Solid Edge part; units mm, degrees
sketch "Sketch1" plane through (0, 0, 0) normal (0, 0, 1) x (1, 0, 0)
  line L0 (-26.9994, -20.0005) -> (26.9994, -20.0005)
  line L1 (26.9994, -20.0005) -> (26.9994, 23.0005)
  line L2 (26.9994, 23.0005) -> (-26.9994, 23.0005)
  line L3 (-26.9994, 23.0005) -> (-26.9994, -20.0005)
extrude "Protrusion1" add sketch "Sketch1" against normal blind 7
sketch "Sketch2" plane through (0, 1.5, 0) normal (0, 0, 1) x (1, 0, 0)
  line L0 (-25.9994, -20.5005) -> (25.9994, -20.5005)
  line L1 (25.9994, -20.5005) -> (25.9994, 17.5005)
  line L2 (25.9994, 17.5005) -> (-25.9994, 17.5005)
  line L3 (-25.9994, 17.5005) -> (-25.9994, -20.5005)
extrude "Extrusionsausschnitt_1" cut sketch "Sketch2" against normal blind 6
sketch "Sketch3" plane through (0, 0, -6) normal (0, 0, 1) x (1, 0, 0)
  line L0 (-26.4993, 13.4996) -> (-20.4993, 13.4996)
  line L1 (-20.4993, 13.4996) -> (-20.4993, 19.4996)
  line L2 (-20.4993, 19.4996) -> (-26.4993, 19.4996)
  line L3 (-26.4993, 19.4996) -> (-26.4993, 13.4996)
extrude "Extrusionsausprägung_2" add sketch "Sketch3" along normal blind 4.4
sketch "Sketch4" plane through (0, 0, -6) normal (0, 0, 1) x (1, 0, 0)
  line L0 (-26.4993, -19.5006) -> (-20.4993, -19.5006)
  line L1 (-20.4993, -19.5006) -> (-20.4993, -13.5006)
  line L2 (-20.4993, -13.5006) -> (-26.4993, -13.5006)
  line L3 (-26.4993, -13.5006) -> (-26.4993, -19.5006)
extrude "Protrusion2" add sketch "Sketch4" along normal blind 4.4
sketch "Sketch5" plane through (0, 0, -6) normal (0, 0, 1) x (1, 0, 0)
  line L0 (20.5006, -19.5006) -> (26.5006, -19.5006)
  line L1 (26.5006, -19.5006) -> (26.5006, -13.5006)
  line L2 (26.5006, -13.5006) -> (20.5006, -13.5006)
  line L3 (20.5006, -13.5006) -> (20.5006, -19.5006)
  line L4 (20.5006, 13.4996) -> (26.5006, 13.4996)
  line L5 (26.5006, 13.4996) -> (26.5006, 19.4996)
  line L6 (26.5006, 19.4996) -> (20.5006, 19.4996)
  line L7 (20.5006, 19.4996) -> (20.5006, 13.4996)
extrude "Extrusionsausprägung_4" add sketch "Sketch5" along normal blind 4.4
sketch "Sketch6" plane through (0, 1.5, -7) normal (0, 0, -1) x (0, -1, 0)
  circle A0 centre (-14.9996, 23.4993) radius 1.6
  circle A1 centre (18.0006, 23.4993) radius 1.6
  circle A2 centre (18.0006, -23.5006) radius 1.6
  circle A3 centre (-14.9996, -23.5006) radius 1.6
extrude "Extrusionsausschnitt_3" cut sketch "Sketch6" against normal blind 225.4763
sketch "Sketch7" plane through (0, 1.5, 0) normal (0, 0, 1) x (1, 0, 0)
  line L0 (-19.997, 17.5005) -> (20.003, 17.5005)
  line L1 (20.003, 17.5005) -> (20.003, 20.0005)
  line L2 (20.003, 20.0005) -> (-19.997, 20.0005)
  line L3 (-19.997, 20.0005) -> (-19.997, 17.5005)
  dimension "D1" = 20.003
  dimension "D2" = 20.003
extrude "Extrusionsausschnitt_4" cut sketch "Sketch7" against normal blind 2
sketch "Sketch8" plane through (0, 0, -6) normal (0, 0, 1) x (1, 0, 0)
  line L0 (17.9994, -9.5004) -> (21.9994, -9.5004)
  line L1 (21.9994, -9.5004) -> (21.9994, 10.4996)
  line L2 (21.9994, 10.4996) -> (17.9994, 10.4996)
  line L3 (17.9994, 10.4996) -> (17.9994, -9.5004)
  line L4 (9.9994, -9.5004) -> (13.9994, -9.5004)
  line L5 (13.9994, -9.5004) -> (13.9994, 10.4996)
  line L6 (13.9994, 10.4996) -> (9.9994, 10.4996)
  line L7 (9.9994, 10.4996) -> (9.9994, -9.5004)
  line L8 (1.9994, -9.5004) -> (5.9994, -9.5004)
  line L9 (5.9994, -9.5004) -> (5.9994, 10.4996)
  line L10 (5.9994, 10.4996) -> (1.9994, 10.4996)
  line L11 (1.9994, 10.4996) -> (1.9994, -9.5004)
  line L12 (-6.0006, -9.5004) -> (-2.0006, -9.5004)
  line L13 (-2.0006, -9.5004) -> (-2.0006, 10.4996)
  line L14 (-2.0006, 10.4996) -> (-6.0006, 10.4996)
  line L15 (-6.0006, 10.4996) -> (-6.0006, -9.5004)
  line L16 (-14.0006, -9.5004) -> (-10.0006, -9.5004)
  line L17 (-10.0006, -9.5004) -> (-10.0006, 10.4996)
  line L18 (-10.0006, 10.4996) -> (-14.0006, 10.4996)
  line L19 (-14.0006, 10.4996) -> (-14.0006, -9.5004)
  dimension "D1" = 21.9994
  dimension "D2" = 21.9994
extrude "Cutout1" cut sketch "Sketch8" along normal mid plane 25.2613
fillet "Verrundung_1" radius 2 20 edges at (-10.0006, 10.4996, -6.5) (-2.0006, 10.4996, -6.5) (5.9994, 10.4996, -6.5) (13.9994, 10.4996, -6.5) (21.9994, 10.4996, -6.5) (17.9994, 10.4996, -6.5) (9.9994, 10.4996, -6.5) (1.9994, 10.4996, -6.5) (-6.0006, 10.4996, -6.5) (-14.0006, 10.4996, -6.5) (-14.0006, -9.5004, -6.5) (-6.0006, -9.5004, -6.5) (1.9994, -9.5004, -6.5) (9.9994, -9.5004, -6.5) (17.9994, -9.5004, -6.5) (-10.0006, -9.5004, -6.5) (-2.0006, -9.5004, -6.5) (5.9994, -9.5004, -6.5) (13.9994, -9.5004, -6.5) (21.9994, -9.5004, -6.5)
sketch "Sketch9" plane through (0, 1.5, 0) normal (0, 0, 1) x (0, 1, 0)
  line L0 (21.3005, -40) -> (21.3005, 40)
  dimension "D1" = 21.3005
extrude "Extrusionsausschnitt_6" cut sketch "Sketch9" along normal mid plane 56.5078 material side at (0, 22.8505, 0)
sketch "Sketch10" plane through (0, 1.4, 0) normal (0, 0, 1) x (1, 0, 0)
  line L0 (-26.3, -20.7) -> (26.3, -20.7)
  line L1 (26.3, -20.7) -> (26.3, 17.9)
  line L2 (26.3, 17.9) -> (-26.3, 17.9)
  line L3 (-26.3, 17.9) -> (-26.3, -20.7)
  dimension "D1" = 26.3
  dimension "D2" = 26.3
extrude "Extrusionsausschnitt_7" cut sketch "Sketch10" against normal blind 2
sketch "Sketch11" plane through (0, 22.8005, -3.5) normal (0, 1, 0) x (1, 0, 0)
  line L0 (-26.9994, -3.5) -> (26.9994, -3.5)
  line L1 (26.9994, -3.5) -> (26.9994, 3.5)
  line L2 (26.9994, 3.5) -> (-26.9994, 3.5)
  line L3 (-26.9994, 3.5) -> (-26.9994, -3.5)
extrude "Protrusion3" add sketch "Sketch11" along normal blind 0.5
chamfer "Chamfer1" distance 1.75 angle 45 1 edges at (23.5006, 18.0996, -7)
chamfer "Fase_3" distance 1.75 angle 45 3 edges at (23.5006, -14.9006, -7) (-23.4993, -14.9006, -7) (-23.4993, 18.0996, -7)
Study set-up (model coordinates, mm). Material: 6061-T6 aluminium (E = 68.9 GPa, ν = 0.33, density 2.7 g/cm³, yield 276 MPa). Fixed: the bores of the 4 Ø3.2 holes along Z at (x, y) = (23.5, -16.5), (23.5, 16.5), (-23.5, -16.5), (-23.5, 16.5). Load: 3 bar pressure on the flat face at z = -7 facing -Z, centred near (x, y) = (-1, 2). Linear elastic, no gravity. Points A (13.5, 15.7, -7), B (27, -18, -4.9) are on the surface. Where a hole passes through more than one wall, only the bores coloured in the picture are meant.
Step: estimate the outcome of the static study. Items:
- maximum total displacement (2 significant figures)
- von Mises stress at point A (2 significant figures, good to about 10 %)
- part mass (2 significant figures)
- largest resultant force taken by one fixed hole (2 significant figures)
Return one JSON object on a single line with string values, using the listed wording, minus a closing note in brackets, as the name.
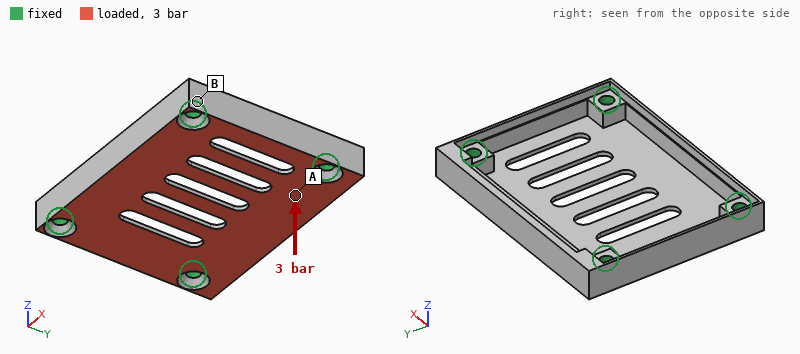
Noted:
{"maximum total displacement": "0.36 mm", "von Mises stress at point A": "66 MPa", "part mass": "11 g", "largest resultant force taken by one fixed hole": "180 N"}
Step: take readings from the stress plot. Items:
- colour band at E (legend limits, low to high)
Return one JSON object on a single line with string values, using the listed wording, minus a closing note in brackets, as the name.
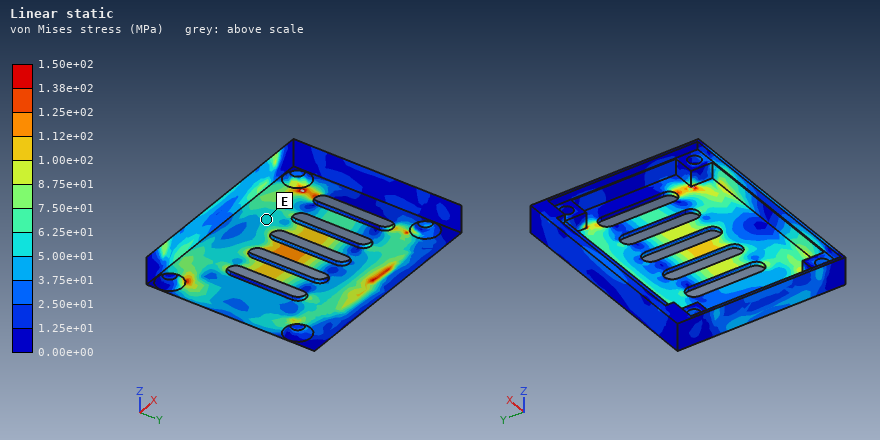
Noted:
{"colour band at E": "5.00e+01 to 6.25e+01 MPa"}
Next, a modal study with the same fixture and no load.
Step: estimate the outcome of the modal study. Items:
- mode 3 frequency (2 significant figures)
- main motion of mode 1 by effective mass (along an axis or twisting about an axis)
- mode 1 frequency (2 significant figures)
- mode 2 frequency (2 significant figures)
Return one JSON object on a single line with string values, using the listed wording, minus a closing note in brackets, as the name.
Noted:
{"mode 3 frequency": "7400 Hz", "main motion of mode 1 by effective mass": "along Z", "mode 1 frequency": "3700 Hz", "mode 2 frequency": "5700 Hz"}
